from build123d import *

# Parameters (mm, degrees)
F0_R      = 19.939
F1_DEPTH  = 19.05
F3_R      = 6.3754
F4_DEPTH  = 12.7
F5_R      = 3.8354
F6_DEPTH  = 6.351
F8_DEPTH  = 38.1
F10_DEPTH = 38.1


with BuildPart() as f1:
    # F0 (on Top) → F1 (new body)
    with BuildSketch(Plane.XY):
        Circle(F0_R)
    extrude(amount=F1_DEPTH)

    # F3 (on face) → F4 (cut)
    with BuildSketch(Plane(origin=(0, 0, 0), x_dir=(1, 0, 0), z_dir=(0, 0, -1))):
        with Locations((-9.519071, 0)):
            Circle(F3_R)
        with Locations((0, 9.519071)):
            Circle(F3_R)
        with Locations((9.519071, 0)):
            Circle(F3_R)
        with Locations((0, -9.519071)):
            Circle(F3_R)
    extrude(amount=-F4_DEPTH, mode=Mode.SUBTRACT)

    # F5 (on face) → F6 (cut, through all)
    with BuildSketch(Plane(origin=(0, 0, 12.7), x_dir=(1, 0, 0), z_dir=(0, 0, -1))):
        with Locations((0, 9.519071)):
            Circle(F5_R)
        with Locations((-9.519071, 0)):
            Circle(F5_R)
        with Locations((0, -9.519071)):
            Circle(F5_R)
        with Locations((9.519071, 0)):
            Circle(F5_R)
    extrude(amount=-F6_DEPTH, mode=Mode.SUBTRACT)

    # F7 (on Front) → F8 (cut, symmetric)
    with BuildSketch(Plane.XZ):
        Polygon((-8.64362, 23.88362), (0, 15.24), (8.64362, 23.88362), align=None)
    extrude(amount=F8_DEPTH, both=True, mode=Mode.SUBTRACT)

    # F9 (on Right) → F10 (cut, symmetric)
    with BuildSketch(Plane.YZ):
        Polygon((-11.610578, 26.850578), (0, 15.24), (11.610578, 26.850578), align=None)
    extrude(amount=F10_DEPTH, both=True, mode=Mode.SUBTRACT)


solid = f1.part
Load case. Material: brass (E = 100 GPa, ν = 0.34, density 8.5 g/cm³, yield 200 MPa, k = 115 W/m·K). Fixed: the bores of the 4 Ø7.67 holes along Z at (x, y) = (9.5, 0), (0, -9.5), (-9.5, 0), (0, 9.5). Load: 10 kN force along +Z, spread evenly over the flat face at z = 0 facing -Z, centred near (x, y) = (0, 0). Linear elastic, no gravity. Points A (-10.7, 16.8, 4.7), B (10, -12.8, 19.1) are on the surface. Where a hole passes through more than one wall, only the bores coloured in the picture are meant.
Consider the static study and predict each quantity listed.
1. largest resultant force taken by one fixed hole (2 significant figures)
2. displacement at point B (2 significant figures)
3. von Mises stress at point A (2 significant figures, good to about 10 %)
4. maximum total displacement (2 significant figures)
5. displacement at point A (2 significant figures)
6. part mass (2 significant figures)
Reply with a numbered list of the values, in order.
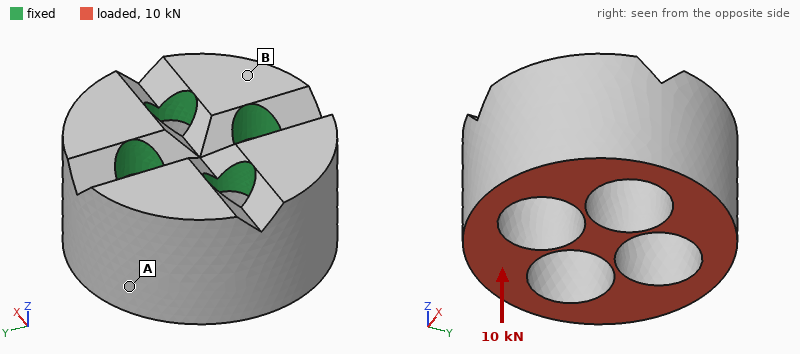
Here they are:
1. 2.5 kN
2. 4.0 µm
3. 15 MPa
4. 6.8 µm
5. 5.8 µm
6. 130 g
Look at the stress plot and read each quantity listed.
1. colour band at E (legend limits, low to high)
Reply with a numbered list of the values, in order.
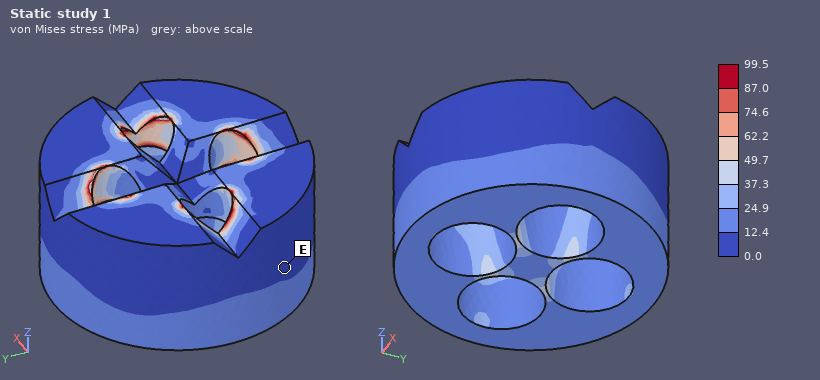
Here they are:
1. 0.0 to 12.4 MPa
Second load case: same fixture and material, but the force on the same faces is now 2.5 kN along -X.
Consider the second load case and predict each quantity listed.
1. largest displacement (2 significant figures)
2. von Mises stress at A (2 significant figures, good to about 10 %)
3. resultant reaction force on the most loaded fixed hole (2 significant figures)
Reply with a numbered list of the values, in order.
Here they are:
1. 8.6 µm
2. 5.9 MPa
3. 1.3 kN
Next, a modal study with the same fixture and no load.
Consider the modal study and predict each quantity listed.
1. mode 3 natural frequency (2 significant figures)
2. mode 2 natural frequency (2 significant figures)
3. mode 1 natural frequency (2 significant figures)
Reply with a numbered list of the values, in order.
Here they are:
1. 16 kHz
2. 14 kHz
3. 14 kHz
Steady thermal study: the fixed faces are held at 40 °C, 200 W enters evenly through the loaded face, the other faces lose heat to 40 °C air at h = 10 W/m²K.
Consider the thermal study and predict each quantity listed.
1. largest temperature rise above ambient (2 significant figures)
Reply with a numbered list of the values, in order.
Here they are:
1. 46 K
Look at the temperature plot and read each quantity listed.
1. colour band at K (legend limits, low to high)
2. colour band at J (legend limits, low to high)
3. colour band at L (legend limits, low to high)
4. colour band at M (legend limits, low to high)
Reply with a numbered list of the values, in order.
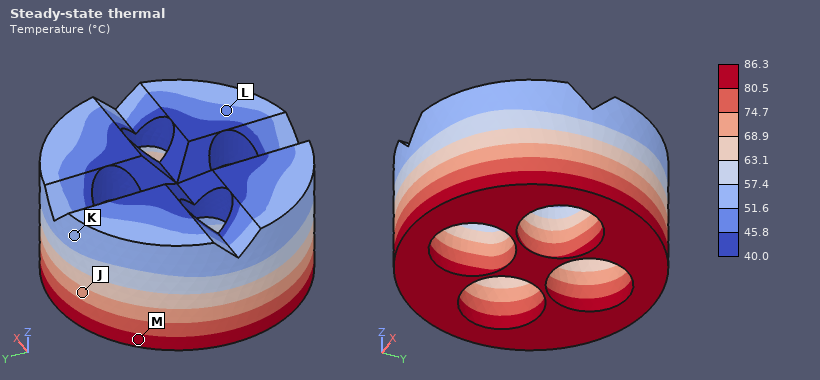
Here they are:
1. 51.6 to 57.4 °C
2. 68.9 to 74.7 °C
3. 45.8 to 51.6 °C
4. 80.5 to 86.3 °C
